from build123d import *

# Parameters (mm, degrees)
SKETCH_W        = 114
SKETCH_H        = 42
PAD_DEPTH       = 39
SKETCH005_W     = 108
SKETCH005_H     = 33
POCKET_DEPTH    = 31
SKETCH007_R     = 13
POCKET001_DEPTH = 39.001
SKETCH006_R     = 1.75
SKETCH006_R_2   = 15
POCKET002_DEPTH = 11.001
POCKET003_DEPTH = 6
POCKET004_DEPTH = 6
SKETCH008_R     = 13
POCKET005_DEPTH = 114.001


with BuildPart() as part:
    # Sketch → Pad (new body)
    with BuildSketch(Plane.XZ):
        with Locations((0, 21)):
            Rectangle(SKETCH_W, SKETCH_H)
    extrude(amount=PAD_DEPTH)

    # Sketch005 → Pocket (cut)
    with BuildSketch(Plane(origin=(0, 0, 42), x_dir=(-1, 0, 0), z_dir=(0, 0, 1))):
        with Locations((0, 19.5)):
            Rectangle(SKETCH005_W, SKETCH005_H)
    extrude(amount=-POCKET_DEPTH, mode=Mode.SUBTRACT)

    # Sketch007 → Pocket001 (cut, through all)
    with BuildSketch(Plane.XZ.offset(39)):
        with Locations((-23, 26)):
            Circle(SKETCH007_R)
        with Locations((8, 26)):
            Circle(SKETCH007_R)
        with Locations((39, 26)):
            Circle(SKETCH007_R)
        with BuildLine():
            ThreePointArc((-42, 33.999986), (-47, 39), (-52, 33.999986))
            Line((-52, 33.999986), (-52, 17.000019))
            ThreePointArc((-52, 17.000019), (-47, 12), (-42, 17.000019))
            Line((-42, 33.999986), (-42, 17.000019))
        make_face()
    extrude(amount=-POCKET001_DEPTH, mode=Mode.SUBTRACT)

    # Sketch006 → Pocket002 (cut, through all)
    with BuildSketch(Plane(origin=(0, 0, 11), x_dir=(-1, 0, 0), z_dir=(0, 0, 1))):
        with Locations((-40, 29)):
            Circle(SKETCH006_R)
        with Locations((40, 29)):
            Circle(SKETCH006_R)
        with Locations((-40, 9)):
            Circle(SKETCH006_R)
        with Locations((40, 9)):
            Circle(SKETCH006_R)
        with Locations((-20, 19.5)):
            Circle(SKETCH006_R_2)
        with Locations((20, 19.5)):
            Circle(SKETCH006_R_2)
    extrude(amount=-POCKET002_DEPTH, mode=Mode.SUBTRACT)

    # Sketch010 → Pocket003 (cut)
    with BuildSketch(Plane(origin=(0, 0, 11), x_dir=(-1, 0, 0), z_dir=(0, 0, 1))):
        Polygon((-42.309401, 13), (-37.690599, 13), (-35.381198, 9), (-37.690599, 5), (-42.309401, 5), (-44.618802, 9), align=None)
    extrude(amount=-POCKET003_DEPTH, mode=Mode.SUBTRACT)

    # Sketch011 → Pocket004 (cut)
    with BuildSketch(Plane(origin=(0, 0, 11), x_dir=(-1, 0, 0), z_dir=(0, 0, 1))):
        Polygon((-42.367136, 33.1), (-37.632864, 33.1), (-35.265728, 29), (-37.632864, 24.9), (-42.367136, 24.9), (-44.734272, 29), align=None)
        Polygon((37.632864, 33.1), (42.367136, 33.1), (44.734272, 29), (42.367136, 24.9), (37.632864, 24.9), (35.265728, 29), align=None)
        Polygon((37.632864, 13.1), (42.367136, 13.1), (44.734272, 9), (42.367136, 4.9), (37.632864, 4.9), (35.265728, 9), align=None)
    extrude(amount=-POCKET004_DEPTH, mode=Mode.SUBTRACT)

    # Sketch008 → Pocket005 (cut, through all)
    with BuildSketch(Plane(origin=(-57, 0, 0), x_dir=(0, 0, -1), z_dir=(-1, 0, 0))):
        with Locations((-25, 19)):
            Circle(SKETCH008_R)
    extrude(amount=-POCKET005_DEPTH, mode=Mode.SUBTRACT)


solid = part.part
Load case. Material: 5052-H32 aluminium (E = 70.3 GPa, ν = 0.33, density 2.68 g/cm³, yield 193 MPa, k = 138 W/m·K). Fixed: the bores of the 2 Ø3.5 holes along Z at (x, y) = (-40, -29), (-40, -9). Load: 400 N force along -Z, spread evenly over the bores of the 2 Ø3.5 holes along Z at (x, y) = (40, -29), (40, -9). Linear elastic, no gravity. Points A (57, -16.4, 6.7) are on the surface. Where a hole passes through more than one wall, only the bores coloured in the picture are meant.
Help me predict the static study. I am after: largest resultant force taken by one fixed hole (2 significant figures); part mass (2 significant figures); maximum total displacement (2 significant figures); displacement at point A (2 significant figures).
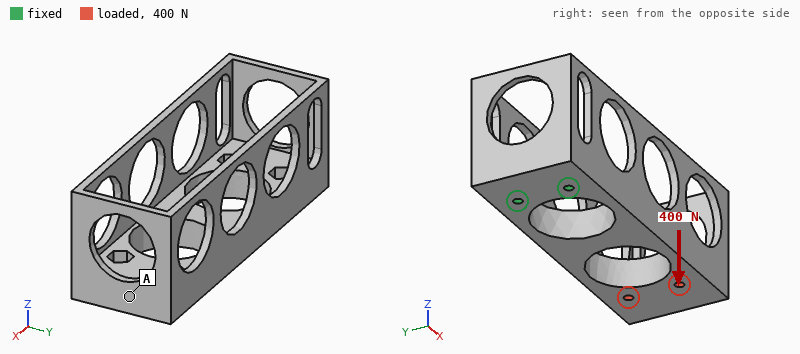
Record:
370 N
120 g
0.56 mm
0.53 mm
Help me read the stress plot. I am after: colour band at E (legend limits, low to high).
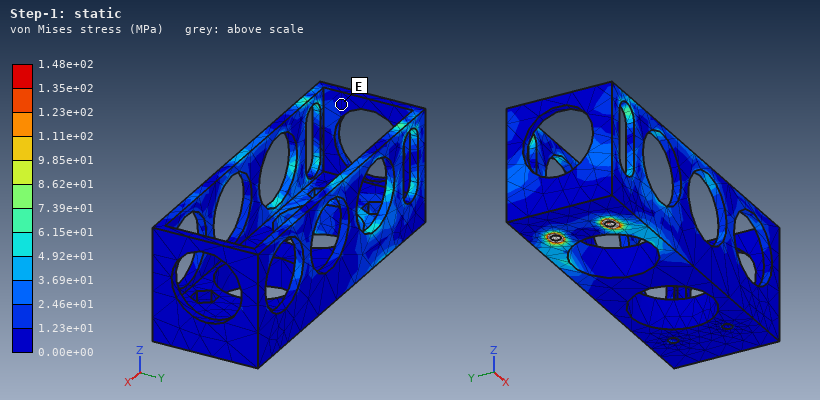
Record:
0.00e+00 to 1.23e+01 MPa
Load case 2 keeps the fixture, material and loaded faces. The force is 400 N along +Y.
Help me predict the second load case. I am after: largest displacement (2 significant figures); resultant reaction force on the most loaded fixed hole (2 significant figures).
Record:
0.11 mm
1.4 kN
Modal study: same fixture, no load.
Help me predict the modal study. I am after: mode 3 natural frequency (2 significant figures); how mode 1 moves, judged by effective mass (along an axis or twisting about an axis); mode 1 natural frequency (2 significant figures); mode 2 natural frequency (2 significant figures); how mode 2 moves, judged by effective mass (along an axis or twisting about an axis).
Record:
1700 Hz
along Z
630 Hz
1300 Hz
along Y
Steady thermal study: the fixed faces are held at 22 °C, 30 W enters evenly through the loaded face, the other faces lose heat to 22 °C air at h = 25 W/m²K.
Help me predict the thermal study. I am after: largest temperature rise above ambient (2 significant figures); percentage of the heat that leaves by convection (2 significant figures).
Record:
60 K
50 %
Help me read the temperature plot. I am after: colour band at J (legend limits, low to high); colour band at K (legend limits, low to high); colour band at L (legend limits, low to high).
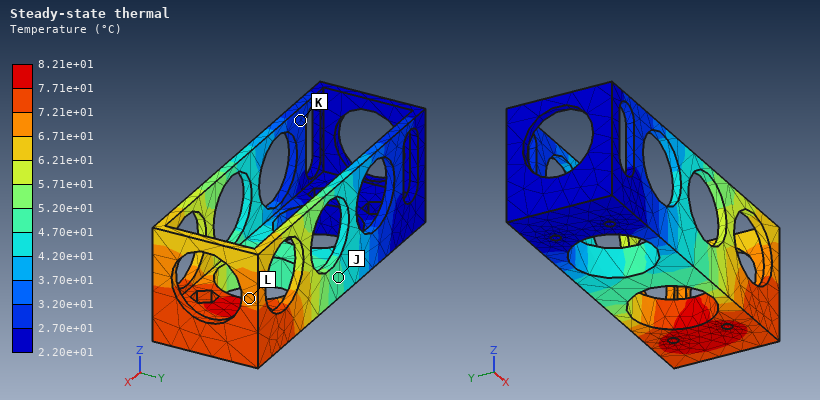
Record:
4.70e+01 to 5.20e+01 °C
2.70e+01 to 3.20e+01 °C
6.71e+01 to 7.21e+01 °C
